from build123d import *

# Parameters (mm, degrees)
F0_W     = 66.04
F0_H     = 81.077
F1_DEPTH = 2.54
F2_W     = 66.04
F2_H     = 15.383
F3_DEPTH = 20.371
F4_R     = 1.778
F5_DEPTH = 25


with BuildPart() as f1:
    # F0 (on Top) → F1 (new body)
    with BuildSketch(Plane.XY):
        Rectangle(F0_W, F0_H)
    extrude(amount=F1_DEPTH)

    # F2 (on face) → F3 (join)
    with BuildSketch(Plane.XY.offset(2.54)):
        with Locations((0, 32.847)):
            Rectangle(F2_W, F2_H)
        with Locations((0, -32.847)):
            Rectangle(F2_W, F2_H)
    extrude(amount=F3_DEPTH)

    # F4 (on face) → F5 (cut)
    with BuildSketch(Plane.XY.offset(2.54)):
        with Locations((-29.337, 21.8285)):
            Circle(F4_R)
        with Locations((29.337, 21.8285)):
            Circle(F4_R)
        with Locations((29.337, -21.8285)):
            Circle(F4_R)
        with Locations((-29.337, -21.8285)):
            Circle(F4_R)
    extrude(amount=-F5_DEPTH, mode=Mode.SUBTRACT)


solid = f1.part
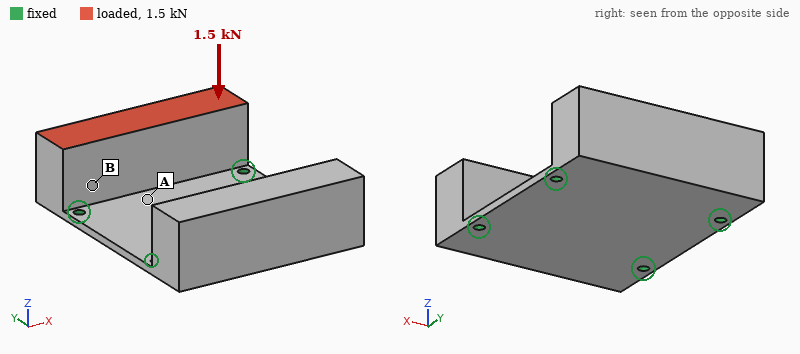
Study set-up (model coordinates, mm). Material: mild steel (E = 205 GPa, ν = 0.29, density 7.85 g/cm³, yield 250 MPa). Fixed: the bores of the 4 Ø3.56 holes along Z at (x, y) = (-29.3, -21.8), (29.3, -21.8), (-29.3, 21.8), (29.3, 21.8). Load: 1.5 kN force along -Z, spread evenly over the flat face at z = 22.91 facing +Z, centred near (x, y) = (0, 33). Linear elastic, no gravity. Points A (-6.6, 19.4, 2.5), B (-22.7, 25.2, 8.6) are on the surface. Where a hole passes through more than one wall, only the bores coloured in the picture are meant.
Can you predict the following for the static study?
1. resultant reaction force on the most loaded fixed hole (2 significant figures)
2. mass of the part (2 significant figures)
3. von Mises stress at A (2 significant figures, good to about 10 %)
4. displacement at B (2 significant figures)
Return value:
830 N
430 g
70 MPa
0.034 mm
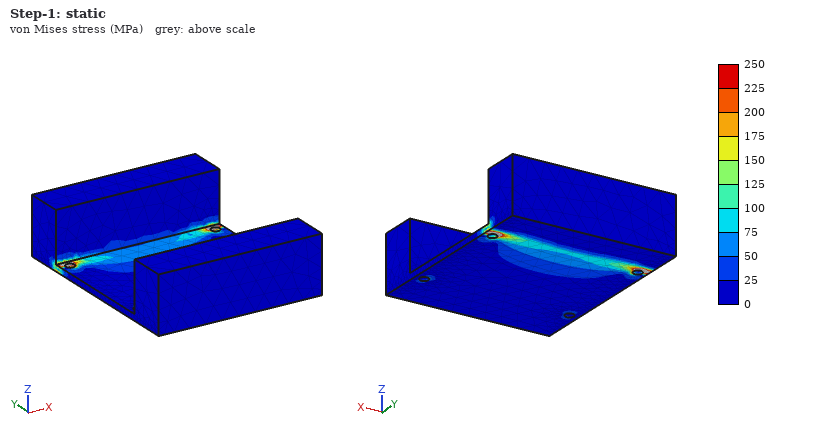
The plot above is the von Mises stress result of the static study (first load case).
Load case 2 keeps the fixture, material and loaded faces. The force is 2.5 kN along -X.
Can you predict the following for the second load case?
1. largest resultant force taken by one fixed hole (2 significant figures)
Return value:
1.5 kN
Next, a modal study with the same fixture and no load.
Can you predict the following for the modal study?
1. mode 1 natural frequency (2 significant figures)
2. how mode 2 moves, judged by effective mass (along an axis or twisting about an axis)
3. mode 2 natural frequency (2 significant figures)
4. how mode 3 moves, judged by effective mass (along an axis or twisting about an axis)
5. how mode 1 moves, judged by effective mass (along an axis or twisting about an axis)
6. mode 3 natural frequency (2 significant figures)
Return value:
1200 Hz
along Y
1300 Hz
along Z
along Z
5400 Hz
